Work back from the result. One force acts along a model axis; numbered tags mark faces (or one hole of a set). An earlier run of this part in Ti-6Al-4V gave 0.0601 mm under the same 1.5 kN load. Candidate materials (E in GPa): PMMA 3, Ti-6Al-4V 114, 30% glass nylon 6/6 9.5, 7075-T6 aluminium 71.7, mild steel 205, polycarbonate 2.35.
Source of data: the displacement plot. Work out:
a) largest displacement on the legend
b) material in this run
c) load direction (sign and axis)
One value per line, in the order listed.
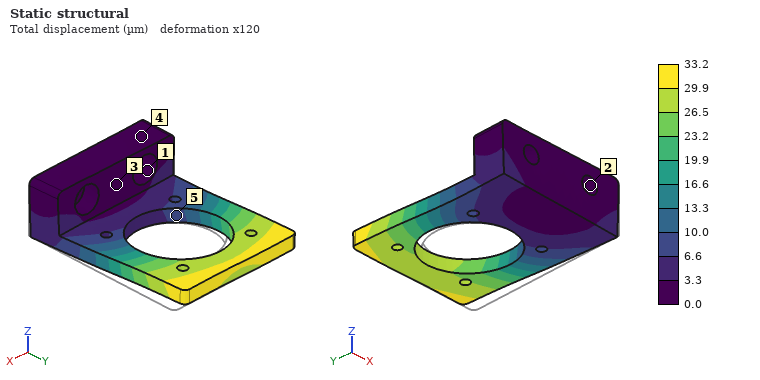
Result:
33.2 µm
mild steel
-X
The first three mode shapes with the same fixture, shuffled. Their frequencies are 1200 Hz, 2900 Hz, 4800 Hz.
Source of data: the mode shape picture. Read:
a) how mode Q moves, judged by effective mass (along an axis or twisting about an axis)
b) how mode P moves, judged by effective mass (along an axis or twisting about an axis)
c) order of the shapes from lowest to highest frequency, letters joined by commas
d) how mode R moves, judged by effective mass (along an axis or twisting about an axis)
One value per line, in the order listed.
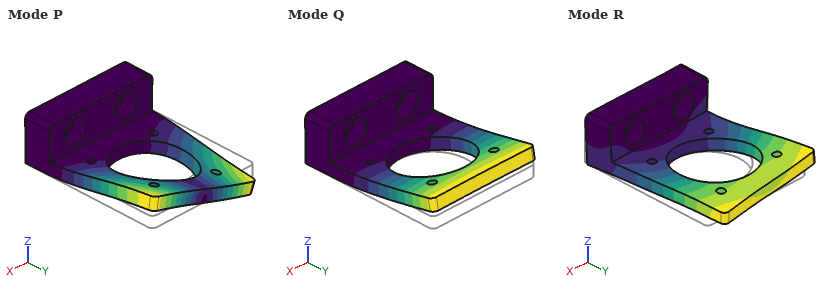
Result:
along Z
twisting about Y
Q, P, R
along X
